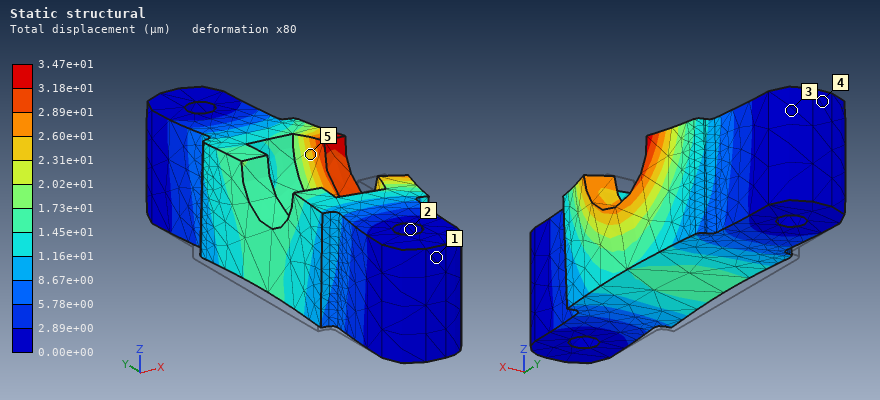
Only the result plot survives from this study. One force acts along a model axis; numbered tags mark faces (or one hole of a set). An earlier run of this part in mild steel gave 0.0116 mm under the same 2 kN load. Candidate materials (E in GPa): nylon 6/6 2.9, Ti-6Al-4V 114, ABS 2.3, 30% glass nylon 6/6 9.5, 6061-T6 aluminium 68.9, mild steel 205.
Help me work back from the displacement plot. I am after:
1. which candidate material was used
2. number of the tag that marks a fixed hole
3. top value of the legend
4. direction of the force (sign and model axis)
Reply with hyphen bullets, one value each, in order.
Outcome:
- 6061-T6 aluminium
- 2
- 3.47e+01 µm
- +X
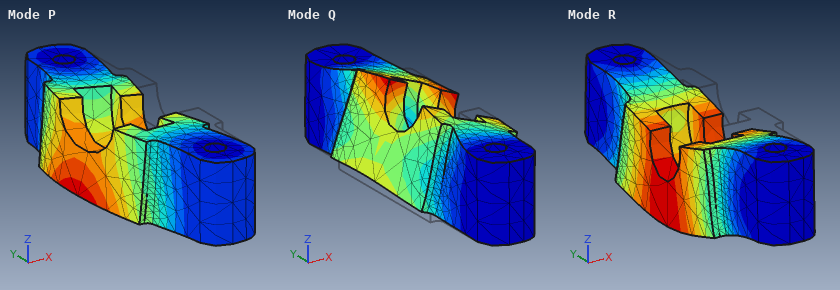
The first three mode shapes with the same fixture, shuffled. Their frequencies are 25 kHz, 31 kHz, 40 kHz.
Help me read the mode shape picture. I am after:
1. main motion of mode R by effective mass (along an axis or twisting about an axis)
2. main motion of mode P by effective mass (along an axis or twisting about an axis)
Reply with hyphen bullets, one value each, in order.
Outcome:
- along Z
- along X
